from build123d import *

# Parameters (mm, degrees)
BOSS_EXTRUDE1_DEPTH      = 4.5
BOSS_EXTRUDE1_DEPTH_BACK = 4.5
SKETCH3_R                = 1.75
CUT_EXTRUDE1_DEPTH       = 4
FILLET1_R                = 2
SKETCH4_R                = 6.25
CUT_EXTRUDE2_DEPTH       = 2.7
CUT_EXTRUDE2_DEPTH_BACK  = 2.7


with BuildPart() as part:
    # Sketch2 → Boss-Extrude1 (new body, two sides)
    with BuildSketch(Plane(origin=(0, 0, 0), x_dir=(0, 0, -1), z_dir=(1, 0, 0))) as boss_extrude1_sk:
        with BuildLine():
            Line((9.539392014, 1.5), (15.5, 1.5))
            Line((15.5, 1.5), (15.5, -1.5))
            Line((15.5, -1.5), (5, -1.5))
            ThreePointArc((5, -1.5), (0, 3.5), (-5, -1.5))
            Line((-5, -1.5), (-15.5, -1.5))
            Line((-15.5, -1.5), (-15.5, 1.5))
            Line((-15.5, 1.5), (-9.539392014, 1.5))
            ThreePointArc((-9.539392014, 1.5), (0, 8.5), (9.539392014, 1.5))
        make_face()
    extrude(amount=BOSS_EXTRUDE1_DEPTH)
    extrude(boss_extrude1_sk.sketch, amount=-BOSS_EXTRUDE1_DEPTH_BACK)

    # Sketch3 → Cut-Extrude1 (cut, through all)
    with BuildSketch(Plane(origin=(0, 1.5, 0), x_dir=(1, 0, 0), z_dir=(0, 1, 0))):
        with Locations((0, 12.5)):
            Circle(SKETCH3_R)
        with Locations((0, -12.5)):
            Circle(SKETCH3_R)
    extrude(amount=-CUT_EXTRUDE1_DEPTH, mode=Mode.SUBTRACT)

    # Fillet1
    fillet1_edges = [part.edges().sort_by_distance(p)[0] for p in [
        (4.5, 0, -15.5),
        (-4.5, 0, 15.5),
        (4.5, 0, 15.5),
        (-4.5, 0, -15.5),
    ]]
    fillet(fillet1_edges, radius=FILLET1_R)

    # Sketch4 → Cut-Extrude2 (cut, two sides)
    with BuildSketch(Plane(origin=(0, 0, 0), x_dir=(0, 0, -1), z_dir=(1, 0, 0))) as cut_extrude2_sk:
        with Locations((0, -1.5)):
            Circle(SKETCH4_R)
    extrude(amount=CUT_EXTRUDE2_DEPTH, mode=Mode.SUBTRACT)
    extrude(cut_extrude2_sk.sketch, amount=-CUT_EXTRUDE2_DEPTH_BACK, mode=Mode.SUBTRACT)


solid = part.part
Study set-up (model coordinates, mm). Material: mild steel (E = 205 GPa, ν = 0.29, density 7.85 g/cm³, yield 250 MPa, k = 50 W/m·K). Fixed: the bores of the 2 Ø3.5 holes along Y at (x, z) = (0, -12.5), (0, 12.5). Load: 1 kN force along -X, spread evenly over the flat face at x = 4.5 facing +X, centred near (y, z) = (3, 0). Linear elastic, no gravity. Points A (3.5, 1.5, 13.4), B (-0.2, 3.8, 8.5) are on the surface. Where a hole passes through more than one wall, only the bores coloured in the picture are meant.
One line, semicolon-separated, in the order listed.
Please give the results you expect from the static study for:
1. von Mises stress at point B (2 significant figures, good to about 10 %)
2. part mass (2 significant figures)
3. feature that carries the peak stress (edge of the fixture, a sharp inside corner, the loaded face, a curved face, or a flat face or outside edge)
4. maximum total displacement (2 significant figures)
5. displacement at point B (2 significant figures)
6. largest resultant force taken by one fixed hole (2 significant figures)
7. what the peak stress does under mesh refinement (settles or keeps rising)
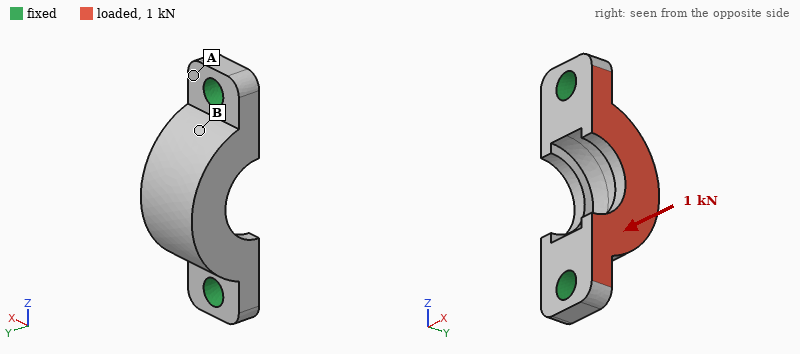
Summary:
42 MPa; 9.2 g; edge of the fixture; 10 µm; 4.2 µm; 500 N; keeps rising
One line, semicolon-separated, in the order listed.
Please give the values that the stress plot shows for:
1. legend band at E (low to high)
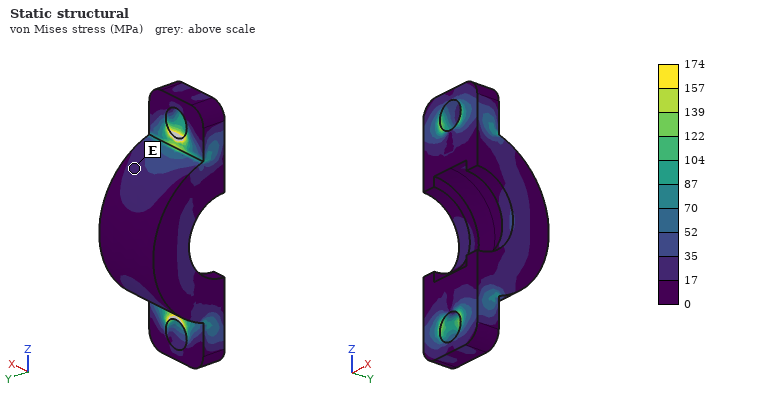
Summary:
17 to 35 MPa
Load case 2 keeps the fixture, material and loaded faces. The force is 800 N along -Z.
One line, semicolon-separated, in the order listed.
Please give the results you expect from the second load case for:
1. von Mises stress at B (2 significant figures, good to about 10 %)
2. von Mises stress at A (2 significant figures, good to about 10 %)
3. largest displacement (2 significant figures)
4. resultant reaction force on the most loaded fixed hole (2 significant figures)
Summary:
11 MPa; 15 MPa; 2.1 µm; 430 N
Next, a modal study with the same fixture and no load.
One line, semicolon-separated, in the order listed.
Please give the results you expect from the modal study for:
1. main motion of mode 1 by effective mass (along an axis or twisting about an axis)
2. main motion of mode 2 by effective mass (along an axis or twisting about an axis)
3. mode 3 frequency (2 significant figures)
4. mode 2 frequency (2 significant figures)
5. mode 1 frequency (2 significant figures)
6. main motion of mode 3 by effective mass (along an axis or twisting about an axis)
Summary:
along X; along Y; 52 kHz; 41 kHz; 20 kHz; along Z
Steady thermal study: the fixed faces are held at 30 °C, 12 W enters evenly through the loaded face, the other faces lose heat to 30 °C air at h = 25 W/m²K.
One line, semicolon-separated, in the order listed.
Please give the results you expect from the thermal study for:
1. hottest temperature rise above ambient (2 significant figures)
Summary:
31 K
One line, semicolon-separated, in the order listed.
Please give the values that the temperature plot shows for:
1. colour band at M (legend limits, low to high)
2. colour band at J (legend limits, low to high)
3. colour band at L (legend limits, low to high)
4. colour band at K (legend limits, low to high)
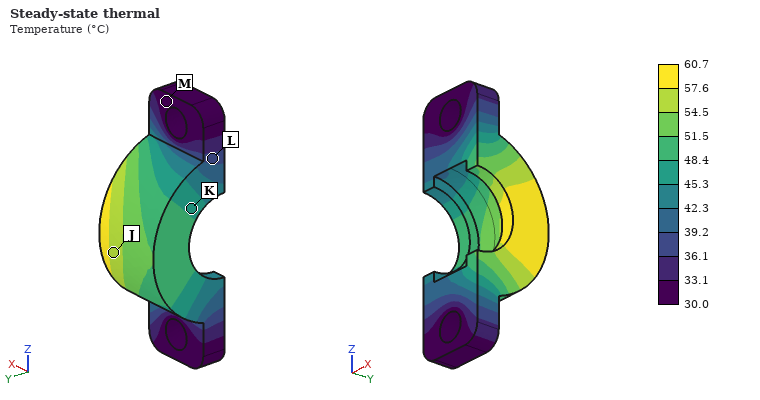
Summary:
30.0 to 33.1 °C; 54.5 to 57.6 °C; 36.1 to 39.2 °C; 45.3 to 48.4 °C
